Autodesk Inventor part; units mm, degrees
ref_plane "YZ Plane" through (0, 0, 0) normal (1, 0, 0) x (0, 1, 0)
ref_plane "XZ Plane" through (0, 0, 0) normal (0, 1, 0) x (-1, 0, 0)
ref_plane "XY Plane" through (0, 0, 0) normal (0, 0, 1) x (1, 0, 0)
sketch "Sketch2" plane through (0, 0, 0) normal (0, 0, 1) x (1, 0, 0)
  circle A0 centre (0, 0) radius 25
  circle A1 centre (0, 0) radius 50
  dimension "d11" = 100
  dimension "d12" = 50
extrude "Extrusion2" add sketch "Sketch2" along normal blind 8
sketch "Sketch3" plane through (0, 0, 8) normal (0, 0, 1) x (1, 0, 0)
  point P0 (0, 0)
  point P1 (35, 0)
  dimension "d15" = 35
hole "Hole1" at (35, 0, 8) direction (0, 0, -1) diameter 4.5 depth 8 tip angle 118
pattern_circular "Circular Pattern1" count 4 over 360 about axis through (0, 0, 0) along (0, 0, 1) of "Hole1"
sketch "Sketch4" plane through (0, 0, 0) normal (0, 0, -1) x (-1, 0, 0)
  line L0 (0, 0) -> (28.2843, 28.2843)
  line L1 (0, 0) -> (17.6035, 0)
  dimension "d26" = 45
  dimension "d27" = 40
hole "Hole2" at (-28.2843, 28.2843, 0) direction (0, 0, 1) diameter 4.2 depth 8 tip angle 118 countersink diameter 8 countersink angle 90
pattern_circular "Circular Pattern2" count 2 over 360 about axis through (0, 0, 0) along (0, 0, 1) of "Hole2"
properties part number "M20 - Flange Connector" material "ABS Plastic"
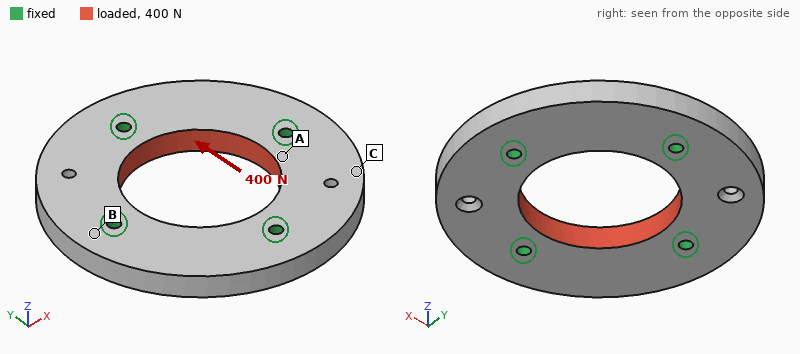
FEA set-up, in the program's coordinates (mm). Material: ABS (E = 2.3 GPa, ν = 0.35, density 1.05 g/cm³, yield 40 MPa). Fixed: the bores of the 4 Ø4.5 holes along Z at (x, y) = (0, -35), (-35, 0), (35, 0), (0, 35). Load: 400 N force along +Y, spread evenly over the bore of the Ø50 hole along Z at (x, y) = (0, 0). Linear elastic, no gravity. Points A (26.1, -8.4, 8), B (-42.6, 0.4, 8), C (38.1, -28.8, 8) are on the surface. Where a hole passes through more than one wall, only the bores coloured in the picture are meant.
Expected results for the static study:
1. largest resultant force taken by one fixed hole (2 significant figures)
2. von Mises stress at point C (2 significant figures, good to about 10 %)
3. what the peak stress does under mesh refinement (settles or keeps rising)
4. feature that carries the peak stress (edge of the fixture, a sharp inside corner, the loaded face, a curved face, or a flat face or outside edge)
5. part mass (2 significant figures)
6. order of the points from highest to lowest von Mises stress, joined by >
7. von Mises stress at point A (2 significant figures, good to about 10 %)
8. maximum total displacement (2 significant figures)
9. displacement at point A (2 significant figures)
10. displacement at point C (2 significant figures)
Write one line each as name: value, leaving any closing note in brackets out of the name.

largest resultant force taken by one fixed hole: 110 N
von Mises stress at point C: 0.24 MPa
what the peak stress does under mesh refinement: keeps rising
feature that carries the peak stress: edge of the fixture
part mass: 49 g
order of the points from highest to lowest von Mises stress, joined by >: A > C > B
von Mises stress at point A: 0.48 MPa
maximum total displacement: 6.8 µm
displacement at point A: 5.1 µm
displacement at point C: 4.0 µm
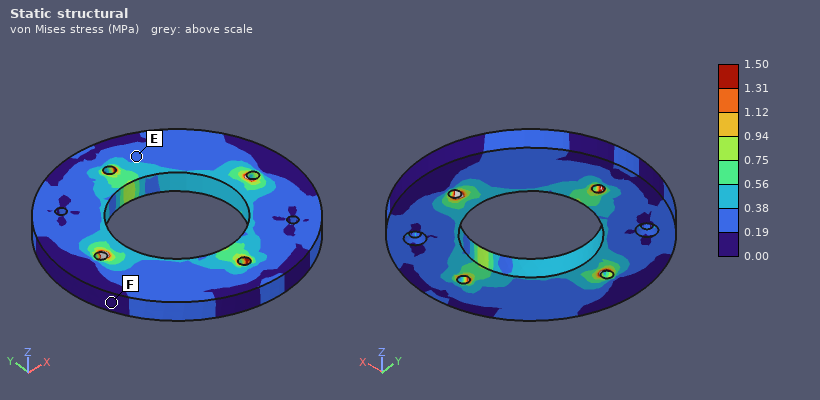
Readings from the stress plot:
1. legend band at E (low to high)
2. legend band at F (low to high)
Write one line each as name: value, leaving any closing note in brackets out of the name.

legend band at E: 0.19 to 0.38 MPa
legend band at F: 0.00 to 0.19 MPa
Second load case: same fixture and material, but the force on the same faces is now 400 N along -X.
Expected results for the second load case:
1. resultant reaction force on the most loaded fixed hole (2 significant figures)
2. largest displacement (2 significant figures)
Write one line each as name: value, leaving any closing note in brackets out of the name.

resultant reaction force on the most loaded fixed hole: 110 N
largest displacement: 6.8 µm
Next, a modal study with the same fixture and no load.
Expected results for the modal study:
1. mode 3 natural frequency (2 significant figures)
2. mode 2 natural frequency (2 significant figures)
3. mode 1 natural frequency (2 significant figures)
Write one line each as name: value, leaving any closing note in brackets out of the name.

mode 3 natural frequency: 2400 Hz
mode 2 natural frequency: 2300 Hz
mode 1 natural frequency: 2100 Hz
